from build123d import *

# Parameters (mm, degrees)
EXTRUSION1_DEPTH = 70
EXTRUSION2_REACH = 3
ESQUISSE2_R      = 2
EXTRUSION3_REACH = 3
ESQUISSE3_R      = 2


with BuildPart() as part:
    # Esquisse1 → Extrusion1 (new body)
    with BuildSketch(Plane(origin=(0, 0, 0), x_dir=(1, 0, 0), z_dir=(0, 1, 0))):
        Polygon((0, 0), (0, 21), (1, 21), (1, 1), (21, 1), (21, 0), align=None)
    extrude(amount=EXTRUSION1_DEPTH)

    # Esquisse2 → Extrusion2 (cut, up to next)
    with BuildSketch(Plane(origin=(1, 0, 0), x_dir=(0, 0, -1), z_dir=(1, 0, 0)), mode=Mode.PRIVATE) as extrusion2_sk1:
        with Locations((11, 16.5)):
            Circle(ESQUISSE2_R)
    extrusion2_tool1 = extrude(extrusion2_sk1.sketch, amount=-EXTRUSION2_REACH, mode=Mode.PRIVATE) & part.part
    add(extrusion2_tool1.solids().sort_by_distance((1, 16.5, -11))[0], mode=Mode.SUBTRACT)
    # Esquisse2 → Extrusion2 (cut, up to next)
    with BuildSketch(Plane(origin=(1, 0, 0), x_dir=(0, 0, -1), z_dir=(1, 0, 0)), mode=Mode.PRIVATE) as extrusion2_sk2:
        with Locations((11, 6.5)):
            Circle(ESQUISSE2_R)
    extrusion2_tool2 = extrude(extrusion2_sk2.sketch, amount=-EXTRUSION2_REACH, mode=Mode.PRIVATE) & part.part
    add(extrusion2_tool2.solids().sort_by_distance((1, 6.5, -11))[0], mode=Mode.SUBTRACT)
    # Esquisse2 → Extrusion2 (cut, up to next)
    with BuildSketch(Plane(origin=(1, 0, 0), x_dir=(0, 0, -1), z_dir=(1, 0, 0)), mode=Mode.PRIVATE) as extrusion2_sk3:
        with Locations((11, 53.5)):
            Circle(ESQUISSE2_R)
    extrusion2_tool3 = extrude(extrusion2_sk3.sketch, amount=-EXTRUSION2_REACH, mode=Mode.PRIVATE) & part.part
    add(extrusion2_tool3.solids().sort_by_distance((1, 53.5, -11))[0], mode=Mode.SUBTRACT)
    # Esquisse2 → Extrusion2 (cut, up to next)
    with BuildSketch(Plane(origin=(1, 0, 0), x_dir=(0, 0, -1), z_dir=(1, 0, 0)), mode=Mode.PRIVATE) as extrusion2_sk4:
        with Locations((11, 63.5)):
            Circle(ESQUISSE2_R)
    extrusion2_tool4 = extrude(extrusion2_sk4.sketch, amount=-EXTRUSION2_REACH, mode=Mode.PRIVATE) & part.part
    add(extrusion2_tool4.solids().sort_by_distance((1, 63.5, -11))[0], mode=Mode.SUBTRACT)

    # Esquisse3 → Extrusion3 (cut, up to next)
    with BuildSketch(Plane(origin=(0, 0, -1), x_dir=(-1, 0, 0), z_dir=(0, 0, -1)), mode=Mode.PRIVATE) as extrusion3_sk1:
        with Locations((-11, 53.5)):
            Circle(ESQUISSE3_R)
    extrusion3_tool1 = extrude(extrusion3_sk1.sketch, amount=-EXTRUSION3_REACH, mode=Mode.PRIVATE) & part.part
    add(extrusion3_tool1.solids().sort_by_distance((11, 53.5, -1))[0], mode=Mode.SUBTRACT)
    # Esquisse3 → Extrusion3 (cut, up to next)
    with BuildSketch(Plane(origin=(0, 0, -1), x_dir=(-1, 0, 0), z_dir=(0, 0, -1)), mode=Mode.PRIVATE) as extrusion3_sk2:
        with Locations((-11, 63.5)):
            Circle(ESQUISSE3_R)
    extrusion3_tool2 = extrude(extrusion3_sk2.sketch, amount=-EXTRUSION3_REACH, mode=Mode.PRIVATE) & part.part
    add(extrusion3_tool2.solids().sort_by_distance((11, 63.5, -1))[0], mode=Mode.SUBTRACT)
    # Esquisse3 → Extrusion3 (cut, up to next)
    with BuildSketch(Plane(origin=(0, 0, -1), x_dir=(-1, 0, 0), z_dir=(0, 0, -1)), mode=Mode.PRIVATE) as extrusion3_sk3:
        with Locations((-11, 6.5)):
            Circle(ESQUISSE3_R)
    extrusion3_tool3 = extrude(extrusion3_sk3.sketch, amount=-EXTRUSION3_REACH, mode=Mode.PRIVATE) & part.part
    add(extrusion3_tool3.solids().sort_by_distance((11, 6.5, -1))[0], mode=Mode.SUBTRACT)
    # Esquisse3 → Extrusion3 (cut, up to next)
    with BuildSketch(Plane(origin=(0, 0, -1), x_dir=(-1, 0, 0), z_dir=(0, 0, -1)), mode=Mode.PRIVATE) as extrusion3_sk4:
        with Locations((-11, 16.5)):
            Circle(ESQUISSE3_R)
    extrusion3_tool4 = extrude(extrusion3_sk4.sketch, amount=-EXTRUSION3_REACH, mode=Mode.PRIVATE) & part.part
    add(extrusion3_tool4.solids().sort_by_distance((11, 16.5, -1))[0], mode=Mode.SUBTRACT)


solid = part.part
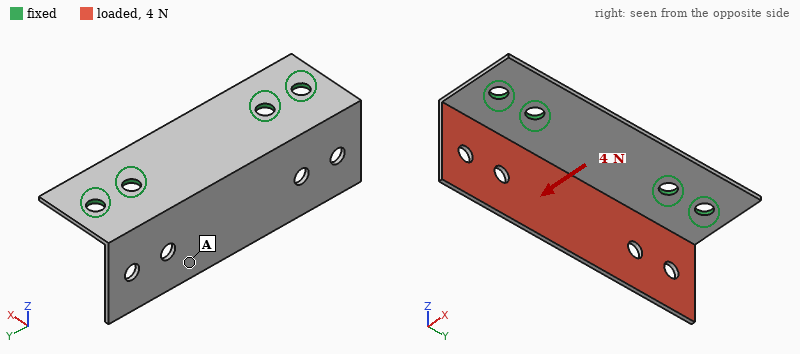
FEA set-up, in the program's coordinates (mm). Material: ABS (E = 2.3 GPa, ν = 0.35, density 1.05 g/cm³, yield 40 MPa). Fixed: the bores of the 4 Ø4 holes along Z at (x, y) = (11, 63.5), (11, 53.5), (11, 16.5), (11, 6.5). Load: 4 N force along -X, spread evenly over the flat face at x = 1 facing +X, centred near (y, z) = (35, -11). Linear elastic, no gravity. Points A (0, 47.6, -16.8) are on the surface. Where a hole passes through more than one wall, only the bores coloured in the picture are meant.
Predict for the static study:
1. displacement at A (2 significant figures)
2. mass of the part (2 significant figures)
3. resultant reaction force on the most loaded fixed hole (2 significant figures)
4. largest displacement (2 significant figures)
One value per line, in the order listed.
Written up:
0.68 mm
2.9 g
1.8 N
0.88 mm
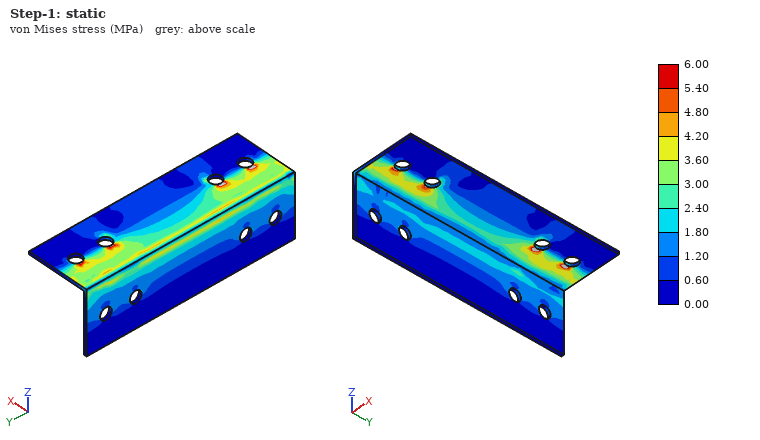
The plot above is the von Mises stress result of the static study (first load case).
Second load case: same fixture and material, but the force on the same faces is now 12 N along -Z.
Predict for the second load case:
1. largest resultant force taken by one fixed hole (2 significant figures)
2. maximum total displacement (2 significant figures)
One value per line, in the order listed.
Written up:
3.4 N
0.80 mm
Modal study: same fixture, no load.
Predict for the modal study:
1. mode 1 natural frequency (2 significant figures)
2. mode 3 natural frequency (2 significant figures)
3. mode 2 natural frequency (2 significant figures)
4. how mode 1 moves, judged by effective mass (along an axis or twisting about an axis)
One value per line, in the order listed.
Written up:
340 Hz
890 Hz
480 Hz
along X
